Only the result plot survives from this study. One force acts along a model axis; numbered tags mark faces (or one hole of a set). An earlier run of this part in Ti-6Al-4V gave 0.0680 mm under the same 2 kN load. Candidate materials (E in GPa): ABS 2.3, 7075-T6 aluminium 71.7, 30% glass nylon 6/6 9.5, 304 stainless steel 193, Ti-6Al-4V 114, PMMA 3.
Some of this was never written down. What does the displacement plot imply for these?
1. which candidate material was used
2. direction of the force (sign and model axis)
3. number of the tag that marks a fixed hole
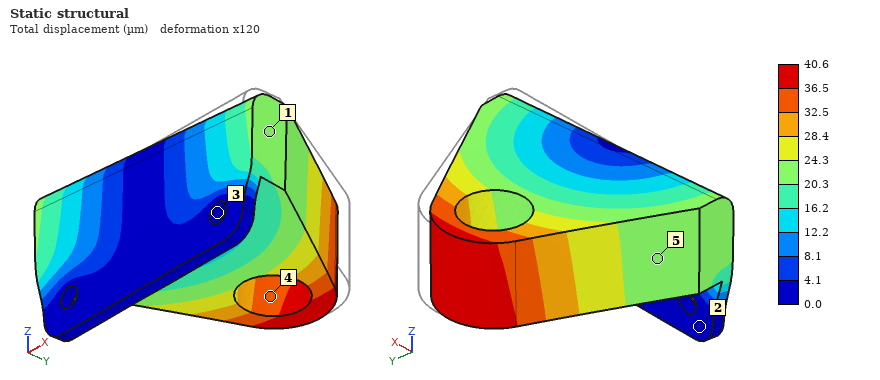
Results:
304 stainless steel
-X
3
